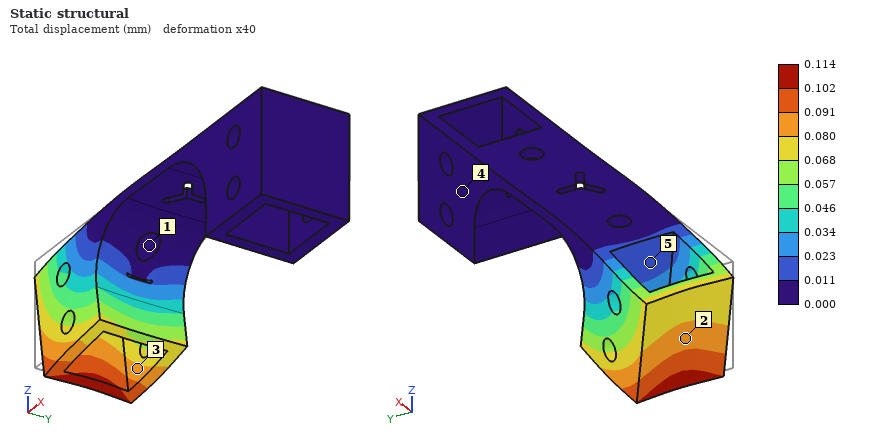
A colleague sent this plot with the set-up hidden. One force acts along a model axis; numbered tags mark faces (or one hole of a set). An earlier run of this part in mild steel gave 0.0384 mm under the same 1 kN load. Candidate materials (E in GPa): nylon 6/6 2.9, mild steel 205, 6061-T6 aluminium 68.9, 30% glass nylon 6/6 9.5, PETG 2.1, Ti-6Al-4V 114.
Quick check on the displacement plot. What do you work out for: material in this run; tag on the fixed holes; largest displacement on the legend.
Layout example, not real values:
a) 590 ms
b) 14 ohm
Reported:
a) 6061-T6 aluminium
b) 1
c) 0.114 mm
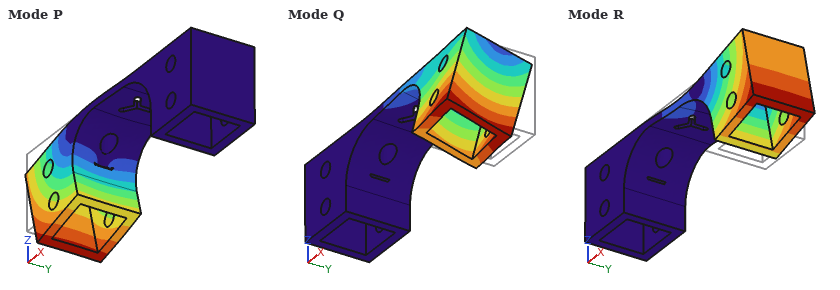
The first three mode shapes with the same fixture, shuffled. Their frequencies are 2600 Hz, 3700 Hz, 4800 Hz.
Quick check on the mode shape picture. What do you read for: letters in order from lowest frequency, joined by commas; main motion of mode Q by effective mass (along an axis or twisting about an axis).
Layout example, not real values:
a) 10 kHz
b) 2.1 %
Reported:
a) R, Q, P
b) along Y
